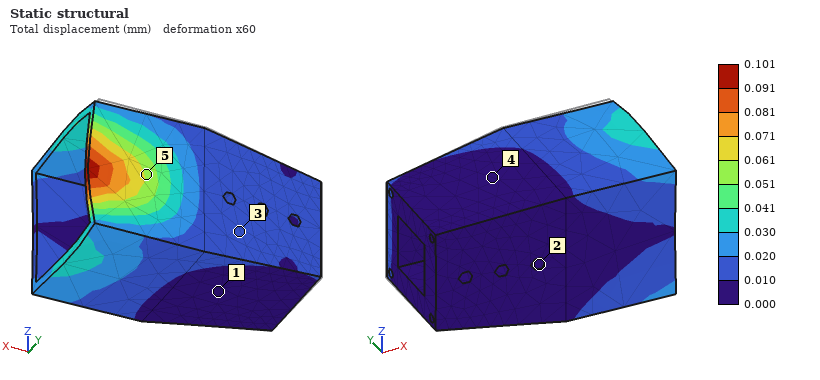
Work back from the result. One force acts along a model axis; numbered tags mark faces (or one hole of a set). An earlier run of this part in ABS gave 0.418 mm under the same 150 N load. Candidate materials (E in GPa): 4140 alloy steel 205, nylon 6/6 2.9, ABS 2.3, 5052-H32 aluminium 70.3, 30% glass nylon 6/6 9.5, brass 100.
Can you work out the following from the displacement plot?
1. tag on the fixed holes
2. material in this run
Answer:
2
30% glass nylon 6/6
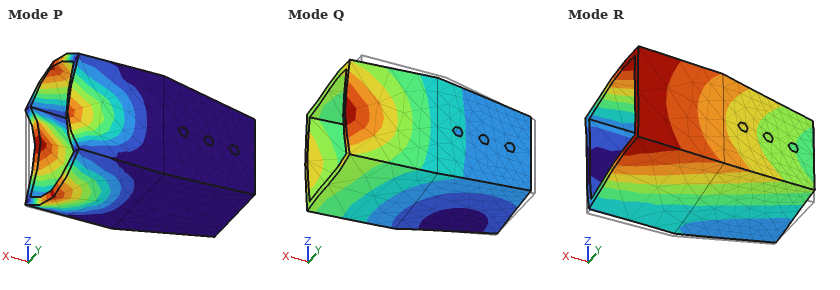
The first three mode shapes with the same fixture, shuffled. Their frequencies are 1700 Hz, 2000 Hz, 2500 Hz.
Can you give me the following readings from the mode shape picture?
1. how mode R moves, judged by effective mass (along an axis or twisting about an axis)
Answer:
along Z
